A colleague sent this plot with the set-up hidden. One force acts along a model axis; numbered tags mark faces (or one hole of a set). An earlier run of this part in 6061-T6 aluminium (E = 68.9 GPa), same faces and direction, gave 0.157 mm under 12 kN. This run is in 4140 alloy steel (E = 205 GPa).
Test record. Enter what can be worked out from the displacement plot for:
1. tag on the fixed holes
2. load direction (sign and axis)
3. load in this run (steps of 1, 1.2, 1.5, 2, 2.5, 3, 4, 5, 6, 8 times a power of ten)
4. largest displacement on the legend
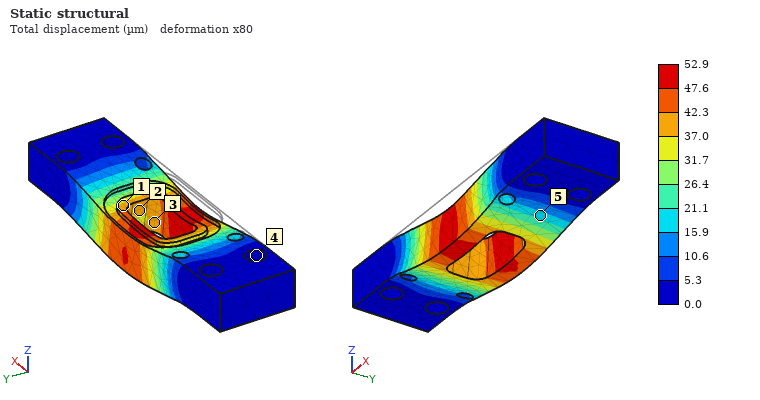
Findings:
4
-Z
12 kN
52.9 µm
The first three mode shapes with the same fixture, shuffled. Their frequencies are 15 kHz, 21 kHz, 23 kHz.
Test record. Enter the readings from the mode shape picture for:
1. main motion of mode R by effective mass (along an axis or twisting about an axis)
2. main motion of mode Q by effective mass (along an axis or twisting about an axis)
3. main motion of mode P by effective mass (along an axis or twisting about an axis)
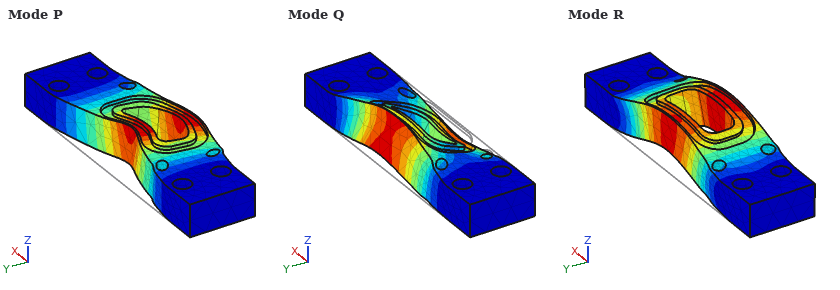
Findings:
along Z
twisting about X
along Y
